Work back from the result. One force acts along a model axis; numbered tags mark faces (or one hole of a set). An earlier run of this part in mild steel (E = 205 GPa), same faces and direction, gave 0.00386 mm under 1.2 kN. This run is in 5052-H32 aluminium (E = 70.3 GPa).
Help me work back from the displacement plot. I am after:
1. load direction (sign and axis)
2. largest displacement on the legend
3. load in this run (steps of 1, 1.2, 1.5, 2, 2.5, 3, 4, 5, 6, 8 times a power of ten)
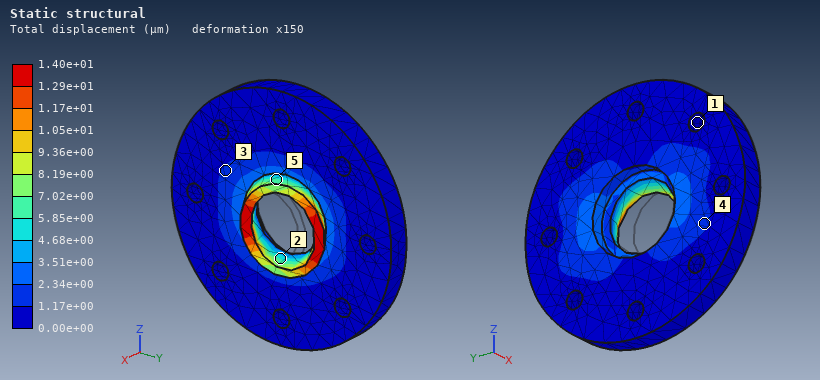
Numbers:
+Y
1.40e+01 µm
1.5 kN
